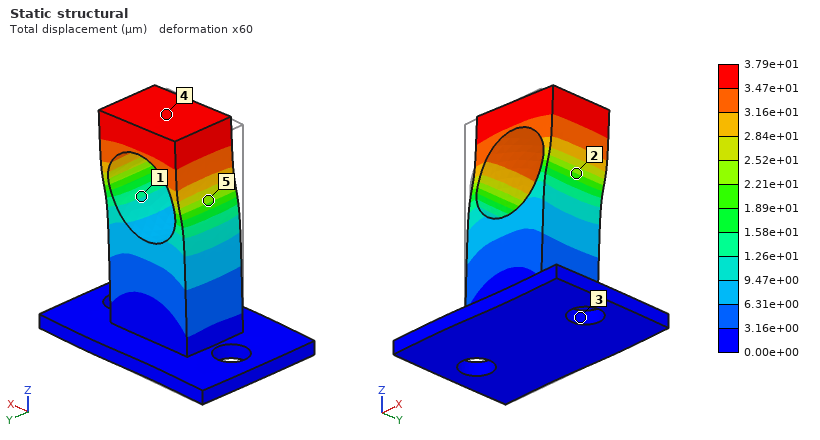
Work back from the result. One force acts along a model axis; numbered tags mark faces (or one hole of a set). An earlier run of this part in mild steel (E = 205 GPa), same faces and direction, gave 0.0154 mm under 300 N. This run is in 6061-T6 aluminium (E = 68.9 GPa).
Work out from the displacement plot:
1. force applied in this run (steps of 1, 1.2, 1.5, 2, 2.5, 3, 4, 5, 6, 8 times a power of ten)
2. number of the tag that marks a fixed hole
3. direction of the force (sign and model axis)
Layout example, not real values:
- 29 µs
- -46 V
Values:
- 250 N
- 3
- +X
